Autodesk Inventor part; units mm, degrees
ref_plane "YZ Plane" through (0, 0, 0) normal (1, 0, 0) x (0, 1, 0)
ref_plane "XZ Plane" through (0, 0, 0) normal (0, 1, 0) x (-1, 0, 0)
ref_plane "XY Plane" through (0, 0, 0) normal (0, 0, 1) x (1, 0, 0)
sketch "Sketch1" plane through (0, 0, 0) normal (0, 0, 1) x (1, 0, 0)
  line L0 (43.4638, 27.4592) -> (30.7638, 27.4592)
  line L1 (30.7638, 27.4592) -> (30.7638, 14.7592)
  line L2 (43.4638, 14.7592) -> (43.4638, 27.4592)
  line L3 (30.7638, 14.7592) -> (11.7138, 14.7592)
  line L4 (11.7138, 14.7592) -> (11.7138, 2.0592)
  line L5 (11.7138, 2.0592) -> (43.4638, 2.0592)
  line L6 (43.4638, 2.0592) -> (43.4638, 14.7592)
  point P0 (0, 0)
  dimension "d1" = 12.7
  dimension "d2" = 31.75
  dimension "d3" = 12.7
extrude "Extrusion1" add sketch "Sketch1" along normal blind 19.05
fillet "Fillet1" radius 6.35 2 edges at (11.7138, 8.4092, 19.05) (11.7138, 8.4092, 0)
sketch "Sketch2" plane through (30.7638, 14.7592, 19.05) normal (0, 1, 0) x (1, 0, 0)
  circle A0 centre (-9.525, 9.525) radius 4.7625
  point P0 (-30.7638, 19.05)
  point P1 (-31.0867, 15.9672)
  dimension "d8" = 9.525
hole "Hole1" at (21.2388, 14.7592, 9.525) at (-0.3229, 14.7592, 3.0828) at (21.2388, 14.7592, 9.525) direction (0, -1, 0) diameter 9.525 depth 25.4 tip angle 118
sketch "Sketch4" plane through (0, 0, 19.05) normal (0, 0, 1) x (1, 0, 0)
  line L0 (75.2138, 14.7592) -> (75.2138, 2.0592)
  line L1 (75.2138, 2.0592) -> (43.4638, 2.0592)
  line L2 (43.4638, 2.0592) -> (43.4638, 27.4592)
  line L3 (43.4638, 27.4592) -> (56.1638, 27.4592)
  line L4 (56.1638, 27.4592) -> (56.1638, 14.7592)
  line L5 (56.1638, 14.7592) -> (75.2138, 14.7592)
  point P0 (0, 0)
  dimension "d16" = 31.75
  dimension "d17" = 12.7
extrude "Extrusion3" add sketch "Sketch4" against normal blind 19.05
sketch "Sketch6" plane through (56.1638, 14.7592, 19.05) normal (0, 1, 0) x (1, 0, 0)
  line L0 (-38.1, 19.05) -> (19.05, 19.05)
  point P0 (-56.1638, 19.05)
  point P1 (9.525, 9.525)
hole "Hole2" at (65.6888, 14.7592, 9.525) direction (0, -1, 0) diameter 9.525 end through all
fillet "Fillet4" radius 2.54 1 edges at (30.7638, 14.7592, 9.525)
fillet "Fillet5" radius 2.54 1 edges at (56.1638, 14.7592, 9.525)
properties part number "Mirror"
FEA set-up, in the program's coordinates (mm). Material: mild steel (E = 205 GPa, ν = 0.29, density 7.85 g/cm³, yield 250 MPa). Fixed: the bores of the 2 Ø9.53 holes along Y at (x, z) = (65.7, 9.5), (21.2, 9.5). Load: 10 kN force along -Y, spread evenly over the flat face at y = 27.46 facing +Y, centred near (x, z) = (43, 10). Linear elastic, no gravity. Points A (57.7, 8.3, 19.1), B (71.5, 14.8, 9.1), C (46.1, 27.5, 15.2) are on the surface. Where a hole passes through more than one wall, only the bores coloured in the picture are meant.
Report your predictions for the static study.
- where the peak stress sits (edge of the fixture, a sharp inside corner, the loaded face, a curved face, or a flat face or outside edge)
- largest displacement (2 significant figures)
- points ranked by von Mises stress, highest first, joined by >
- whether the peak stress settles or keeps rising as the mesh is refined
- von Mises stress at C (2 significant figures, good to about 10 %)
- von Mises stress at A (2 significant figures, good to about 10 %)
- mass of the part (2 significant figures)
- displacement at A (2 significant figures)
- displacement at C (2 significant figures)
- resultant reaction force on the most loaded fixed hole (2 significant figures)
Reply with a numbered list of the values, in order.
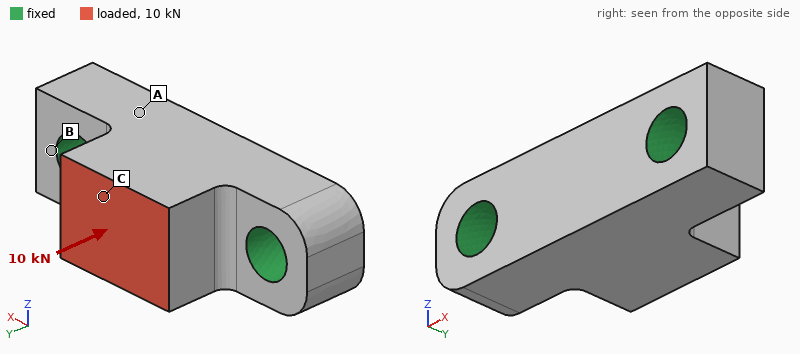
1. edge of the fixture
2. 5.2 µm
3. A > C > B
4. keeps rising
5. 18 MPa
6. 36 MPa
7. 150 g
8. 2.0 µm
9. 5.1 µm
10. 5.3 kN
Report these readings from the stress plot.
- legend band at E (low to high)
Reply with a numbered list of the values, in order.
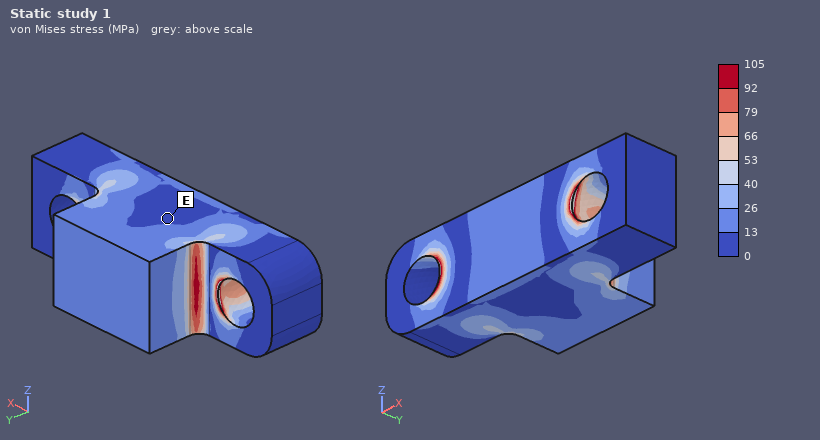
1. 0 to 13 MPa
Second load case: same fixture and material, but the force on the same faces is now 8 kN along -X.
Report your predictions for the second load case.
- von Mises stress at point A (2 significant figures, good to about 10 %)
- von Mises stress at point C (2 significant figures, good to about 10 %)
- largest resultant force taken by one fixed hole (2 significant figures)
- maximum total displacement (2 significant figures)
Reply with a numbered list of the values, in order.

1. 27 MPa
2. 30 MPa
3. 5.9 kN
4. 9.6 µm
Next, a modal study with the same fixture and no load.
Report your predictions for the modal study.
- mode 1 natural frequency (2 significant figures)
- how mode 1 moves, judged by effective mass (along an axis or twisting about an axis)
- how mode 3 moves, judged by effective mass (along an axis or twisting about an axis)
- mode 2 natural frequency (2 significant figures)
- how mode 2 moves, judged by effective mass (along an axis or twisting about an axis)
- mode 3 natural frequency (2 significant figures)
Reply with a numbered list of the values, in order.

1. 15 kHz
2. along Z
3. along Z
4. 25 kHz
5. along Y
6. 31 kHz
